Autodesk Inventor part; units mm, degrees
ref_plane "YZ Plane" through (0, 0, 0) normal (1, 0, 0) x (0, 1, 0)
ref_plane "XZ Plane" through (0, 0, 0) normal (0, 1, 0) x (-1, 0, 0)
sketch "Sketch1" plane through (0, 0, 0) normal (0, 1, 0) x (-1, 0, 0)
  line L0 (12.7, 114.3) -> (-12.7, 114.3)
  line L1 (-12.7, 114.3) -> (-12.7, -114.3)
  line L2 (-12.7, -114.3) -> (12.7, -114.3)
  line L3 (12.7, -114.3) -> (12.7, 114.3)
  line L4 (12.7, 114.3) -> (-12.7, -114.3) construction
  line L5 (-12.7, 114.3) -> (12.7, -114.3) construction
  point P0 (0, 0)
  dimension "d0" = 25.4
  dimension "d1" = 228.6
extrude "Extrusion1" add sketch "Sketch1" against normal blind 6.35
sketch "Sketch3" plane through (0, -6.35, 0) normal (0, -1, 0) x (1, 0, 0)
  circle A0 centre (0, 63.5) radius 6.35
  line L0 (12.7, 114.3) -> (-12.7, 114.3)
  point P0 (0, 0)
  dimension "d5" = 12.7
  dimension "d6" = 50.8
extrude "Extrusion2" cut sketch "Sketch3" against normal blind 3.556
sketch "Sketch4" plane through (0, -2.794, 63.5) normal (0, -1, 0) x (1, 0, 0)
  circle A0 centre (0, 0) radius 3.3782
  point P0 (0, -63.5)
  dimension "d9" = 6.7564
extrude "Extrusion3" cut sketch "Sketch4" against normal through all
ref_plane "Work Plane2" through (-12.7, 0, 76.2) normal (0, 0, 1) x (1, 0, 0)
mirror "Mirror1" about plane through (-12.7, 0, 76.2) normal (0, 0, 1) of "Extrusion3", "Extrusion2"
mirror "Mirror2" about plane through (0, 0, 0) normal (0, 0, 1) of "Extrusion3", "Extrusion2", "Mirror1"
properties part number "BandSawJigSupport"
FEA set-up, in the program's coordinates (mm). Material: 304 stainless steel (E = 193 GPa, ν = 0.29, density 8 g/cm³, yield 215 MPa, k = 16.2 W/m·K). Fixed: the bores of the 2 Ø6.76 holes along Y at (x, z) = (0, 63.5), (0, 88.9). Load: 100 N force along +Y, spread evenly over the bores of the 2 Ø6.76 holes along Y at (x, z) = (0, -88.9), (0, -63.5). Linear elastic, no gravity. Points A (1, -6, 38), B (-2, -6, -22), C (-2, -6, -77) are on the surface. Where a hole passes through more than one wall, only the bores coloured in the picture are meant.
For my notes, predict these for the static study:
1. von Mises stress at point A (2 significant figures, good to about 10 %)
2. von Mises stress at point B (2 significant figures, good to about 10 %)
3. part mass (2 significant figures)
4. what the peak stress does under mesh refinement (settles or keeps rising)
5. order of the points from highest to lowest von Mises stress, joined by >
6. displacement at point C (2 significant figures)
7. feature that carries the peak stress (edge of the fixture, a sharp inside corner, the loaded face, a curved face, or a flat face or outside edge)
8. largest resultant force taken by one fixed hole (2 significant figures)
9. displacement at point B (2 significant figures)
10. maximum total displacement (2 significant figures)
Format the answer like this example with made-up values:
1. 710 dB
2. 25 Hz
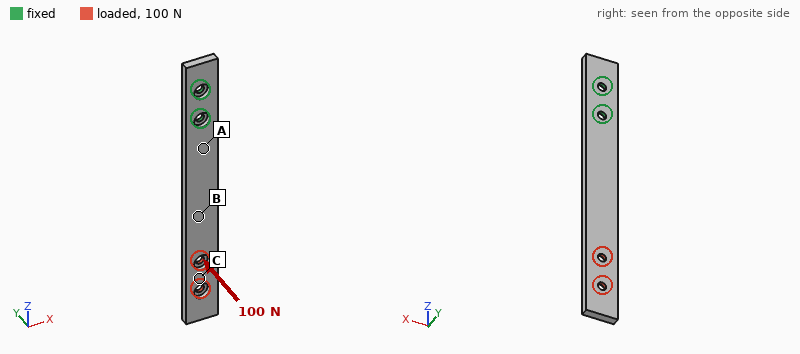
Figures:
1. 65 MPa
2. 32 MPa
3. 280 g
4. keeps rising
5. A > B > C
6. 1.00 mm
7. edge of the fixture
8. 960 N
9. 0.46 mm
10. 1.4 mm
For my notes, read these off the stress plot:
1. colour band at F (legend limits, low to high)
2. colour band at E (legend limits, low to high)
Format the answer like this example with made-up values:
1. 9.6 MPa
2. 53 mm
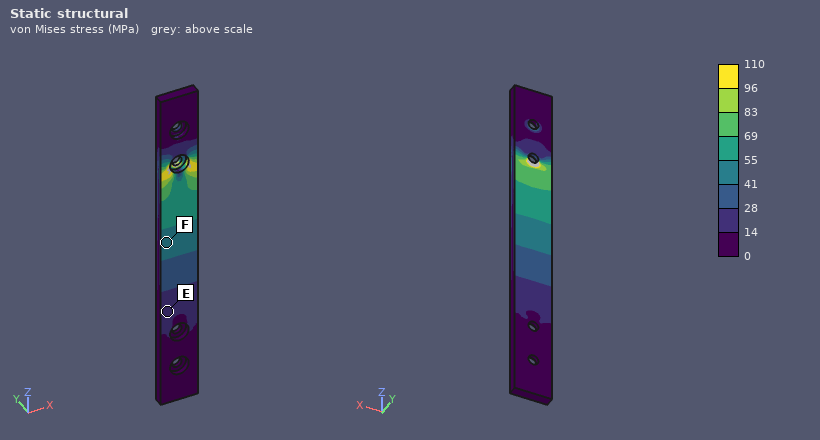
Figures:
1. 41 to 55 MPa
2. 14 to 28 MPa
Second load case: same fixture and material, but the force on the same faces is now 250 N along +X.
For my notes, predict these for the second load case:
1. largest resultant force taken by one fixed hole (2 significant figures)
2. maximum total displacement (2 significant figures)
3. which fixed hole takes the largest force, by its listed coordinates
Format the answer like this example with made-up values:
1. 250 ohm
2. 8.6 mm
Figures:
1. 1.2 kN
2. 0.25 mm
3. (0, 63.5)
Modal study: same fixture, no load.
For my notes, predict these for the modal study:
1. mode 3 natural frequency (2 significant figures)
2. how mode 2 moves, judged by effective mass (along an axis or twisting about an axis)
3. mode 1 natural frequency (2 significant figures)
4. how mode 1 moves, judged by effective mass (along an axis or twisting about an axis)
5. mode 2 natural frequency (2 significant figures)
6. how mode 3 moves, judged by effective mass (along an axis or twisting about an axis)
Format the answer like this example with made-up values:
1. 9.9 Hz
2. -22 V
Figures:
1. 930 Hz
2. along X
3. 160 Hz
4. along Y
5. 570 Hz
6. along Y
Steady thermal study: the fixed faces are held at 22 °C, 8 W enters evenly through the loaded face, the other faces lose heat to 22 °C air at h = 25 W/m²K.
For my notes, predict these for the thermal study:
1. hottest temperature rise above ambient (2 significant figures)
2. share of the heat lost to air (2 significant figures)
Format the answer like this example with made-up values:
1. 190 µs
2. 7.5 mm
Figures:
1. 69 K
2. 97 %
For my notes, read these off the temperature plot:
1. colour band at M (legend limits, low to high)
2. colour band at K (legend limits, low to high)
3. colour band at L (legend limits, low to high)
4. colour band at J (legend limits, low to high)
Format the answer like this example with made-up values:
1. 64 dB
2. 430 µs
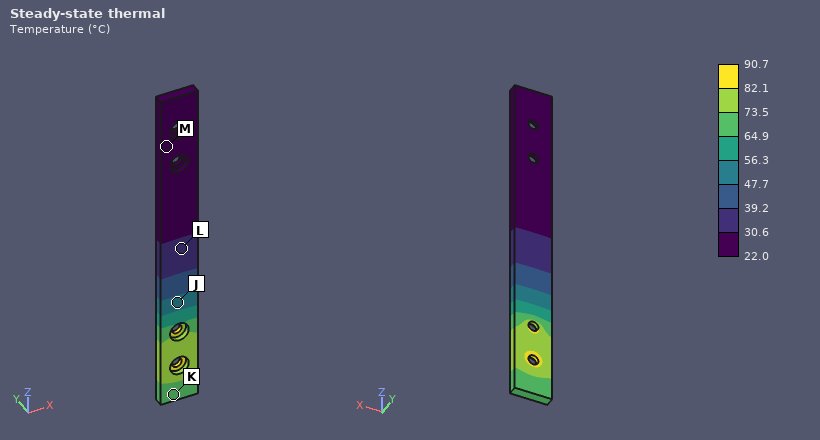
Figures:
1. 22.0 to 30.6 °C
2. 64.9 to 73.5 °C
3. 30.6 to 39.2 °C
4. 47.7 to 56.3 °C
